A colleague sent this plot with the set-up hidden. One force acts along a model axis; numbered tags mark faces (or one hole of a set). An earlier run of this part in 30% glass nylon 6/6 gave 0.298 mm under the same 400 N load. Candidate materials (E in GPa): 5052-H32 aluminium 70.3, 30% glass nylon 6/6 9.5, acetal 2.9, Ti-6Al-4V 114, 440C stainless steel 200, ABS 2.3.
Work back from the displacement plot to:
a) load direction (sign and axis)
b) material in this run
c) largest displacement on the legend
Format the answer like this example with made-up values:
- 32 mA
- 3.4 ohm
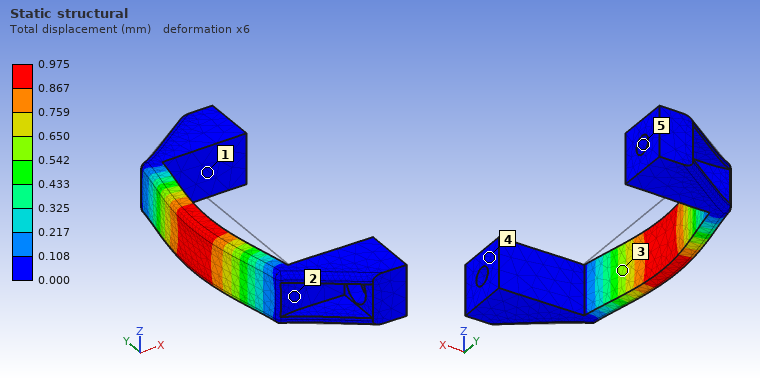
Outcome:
- -X
- acetal
- 0.975 mm
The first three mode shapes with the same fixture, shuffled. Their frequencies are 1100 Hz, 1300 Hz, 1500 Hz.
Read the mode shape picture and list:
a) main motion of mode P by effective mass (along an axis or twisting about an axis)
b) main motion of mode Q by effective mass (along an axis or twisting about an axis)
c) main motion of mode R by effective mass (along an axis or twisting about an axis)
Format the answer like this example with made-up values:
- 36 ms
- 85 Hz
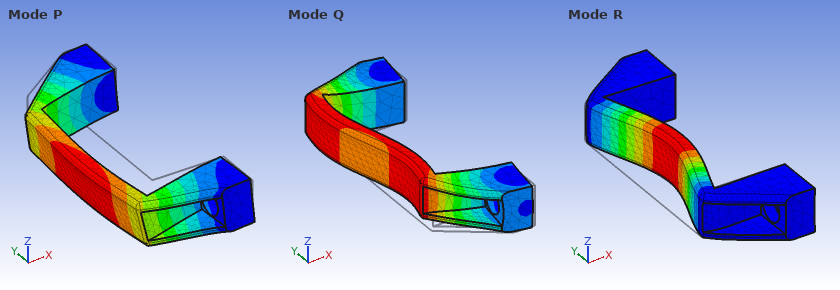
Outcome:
- along Z
- along Y
- along X
